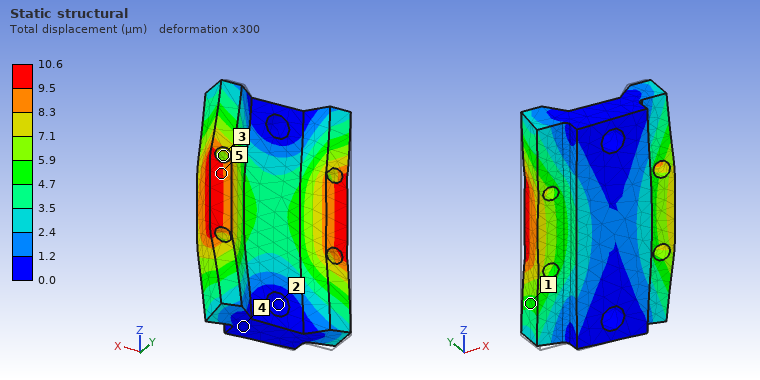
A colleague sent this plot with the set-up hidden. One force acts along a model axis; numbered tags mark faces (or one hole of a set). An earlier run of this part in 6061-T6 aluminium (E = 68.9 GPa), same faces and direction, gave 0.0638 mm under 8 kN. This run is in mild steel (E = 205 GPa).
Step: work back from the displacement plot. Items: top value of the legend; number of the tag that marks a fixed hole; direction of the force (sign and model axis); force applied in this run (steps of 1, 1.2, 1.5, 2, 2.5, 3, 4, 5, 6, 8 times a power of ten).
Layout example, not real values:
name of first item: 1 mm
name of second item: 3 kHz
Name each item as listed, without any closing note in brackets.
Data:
top value of the legend: 10.6 µm
number of the tag that marks a fixed hole: 2
direction of the force: +X
force applied in this run: 4 kN
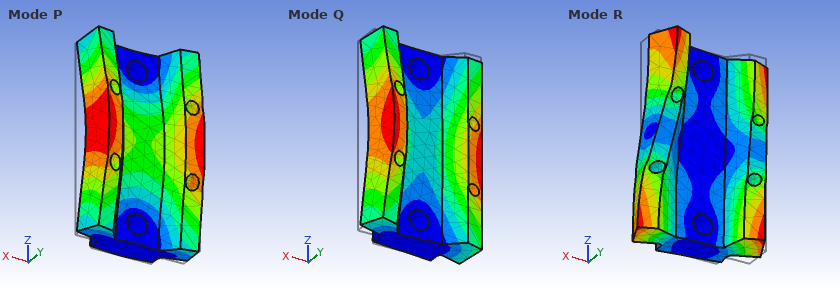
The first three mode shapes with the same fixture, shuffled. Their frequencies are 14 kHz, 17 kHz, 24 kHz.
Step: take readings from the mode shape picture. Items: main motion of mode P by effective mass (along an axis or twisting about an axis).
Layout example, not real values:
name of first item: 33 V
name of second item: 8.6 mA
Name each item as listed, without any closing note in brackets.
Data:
main motion of mode P by effective mass: along Y
